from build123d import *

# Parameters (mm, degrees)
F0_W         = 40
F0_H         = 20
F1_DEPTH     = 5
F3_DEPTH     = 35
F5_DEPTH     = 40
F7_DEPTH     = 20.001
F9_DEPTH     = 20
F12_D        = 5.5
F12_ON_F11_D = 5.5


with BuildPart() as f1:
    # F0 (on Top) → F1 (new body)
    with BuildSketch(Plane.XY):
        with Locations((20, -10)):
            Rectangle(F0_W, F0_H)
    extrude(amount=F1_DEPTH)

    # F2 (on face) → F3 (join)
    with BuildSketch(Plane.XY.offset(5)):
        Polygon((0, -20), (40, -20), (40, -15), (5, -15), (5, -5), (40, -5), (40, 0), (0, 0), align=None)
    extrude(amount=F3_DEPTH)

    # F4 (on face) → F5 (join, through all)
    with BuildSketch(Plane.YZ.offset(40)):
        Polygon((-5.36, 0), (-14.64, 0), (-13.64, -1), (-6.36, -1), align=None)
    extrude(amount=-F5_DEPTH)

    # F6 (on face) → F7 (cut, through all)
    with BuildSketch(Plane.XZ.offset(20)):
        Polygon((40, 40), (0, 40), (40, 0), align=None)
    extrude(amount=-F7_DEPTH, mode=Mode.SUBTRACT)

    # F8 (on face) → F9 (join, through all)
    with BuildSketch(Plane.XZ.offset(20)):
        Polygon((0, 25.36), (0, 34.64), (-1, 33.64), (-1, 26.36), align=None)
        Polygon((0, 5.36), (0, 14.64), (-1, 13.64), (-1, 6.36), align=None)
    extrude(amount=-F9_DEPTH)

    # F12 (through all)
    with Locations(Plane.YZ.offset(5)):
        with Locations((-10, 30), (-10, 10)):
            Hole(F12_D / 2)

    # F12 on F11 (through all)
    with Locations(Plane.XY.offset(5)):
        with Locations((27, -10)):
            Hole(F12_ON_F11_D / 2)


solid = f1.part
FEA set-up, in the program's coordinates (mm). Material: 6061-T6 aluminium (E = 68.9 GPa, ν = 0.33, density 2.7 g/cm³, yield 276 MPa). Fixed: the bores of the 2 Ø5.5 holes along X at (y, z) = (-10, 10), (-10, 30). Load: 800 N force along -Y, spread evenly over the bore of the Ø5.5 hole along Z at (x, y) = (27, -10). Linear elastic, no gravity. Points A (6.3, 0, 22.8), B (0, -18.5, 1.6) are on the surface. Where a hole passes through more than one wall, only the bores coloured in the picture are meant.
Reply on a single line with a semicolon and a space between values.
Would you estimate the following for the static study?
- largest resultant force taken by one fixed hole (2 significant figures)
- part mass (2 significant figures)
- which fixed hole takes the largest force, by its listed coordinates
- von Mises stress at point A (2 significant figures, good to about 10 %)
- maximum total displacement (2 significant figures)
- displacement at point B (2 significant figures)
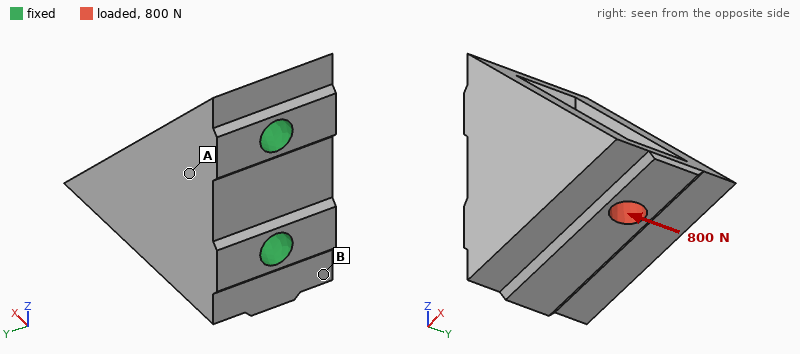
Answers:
930 N; 32 g; (-10, 10); 22 MPa; 74 µm; 14 µm
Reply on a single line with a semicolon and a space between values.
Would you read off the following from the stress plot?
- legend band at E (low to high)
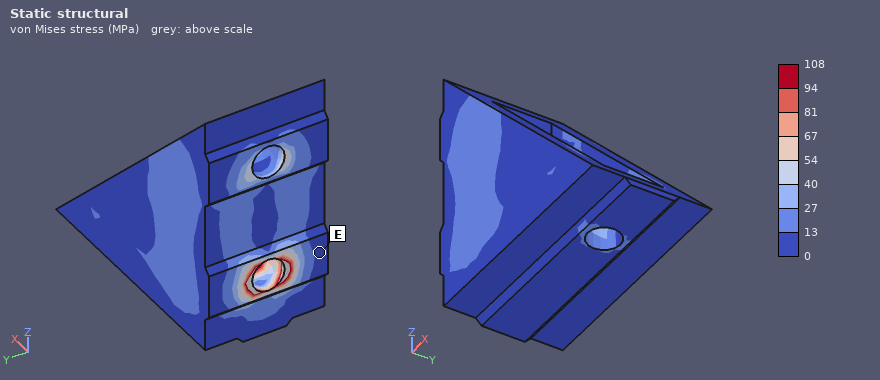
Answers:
0 to 13 MPa
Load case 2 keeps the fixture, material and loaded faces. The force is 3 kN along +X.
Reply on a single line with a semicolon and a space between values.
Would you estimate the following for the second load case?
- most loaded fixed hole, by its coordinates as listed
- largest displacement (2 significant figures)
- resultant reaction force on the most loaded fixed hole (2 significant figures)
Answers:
(-10, 10); 46 µm; 3.7 kN
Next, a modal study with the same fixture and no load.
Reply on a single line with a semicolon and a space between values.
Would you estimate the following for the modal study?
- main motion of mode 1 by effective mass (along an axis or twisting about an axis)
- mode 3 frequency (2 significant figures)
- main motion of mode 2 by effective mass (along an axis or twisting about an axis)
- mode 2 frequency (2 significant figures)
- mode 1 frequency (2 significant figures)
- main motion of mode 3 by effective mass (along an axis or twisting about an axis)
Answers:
along Y; 19 kHz; along Z; 11 kHz; 5800 Hz; along X
